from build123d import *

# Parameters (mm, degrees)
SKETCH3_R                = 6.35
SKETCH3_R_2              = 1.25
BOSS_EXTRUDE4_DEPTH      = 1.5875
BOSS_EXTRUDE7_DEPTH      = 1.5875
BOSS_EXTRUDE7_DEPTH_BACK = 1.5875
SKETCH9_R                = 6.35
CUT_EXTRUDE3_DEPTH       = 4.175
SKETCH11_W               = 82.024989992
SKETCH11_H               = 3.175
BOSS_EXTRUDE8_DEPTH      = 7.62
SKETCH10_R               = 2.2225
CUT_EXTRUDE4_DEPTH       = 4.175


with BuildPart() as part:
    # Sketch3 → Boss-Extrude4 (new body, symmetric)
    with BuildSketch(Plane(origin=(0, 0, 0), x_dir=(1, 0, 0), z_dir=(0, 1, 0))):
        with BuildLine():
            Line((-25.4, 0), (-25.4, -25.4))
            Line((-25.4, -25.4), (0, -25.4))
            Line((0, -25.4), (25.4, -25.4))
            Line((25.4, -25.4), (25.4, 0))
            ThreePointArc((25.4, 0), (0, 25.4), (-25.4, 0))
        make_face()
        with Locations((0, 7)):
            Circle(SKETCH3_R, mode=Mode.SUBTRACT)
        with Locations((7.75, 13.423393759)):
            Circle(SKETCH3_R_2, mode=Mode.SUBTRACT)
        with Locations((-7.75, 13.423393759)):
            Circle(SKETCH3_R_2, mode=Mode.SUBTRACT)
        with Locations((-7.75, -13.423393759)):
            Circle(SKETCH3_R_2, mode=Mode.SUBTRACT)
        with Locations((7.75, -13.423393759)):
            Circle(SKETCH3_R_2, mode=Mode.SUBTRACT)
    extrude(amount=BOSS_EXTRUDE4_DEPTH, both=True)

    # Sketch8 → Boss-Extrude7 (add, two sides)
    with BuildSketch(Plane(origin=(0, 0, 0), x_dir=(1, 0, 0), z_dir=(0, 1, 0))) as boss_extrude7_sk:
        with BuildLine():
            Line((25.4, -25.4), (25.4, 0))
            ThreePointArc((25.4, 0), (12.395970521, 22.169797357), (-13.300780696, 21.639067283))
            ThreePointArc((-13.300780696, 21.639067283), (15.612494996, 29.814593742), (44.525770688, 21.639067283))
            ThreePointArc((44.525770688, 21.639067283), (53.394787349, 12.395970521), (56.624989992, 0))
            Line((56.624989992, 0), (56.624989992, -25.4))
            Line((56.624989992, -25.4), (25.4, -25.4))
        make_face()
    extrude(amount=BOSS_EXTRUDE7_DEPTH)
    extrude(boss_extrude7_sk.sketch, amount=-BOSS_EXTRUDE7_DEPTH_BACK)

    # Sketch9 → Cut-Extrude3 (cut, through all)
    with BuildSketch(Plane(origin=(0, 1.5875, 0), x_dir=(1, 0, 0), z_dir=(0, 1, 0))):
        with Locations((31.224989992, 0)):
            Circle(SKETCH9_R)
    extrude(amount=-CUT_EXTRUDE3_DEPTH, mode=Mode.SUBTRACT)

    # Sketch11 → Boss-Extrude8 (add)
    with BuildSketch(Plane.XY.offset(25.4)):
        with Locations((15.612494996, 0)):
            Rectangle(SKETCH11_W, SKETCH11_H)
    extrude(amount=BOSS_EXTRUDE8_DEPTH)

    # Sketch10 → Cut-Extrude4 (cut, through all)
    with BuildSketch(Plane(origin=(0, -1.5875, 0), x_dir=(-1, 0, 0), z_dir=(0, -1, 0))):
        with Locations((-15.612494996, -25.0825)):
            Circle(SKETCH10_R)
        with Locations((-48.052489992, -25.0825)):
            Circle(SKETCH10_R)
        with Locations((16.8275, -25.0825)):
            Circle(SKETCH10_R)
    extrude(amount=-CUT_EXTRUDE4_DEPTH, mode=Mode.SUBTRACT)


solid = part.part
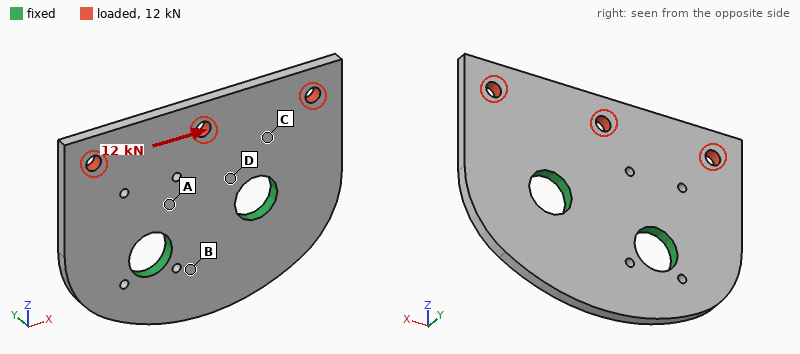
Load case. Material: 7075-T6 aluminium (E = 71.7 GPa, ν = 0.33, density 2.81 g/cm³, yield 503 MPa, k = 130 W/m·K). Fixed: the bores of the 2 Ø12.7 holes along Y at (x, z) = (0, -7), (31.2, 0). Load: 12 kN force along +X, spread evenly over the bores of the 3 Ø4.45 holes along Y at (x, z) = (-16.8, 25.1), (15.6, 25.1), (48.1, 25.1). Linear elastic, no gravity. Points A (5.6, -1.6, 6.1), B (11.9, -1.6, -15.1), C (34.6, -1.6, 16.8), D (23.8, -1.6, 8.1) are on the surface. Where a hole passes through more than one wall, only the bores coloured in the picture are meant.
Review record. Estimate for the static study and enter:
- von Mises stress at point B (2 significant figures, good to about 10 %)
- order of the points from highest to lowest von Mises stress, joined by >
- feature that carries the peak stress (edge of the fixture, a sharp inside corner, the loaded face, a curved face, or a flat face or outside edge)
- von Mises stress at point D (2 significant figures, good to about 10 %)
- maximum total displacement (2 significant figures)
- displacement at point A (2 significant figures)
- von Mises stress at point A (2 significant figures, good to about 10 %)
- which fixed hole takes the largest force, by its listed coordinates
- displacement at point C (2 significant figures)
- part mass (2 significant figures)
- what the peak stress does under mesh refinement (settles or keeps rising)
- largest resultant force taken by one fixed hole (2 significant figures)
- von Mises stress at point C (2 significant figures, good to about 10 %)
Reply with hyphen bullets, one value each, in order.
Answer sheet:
- 24 MPa
- D > A > C > B
- edge of the fixture
- 170 MPa
- 0.12 mm
- 0.020 mm
- 120 MPa
- (31.2, 0)
- 0.049 mm
- 39 g
- keeps rising
- 11 kN
- 94 MPa
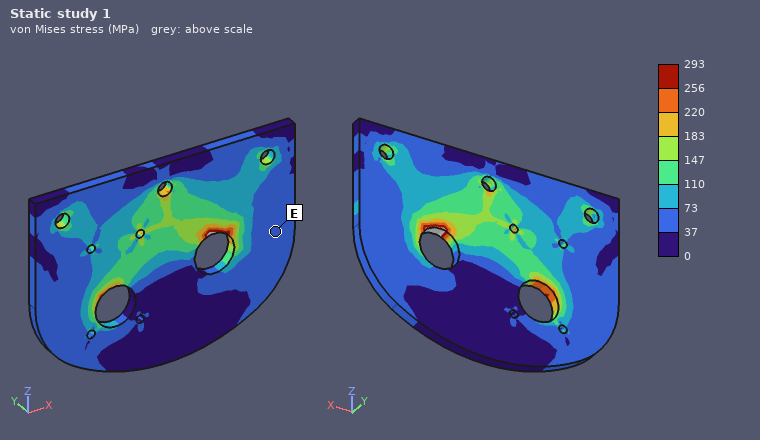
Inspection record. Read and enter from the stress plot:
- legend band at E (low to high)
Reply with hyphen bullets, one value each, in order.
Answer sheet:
- 37 to 73 MPa
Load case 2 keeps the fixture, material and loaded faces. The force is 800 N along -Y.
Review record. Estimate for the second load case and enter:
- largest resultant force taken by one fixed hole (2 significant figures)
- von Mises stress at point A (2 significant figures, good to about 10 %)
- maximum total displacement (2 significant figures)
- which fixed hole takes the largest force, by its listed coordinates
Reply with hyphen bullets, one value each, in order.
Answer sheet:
- 470 N
- 92 MPa
- 0.60 mm
- (31.2, 0)
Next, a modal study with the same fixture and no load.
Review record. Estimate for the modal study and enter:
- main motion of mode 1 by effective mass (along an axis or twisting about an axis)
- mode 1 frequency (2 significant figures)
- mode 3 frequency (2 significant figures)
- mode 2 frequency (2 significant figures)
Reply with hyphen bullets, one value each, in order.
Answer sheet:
- along Y
- 2200 Hz
- 4400 Hz
- 3100 Hz
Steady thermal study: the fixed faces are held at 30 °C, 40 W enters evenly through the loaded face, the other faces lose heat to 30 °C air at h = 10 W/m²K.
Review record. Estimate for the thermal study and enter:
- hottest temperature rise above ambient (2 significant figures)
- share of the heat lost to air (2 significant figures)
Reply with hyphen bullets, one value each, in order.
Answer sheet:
- 45 K
- 3.4 %
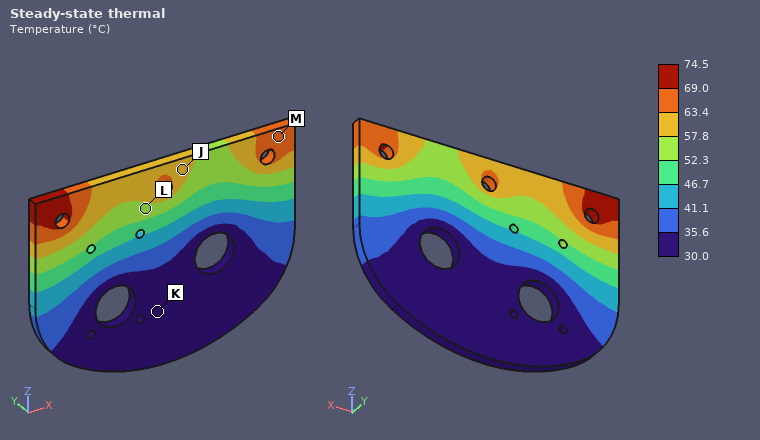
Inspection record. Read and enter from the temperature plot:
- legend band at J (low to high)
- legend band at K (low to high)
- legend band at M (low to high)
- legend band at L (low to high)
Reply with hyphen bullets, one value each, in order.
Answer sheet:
- 57.8 to 63.4 °C
- 30.0 to 35.6 °C
- 63.4 to 69.0 °C
- 52.3 to 57.8 °C
